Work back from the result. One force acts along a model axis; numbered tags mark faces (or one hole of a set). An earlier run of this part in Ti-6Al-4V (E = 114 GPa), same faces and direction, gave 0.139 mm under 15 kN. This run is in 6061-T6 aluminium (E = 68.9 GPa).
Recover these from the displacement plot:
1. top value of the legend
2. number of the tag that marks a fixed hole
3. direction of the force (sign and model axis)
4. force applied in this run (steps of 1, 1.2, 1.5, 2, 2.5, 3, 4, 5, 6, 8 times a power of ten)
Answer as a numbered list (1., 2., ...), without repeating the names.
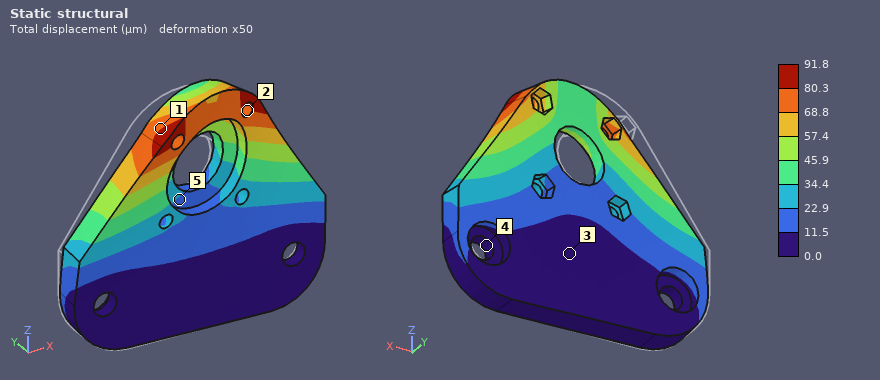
1. 91.8 µm
2. 4
3. +X
4. 6 kN
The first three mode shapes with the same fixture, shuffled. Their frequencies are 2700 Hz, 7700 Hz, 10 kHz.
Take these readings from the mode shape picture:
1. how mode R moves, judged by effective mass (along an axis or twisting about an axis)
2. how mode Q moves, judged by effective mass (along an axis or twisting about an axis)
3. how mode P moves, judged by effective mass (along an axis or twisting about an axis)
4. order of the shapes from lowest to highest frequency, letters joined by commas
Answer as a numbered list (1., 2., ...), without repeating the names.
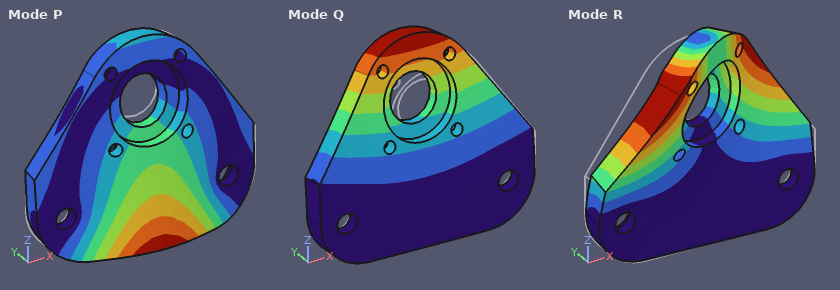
1. twisting about Z
2. along Y
3. along Y
4. Q, R, P
